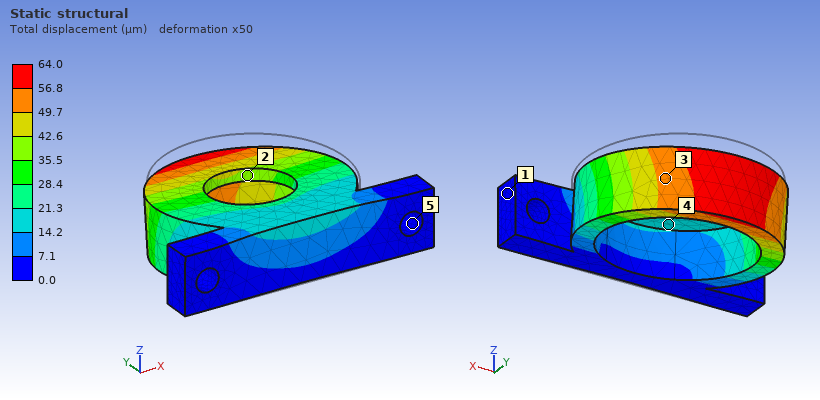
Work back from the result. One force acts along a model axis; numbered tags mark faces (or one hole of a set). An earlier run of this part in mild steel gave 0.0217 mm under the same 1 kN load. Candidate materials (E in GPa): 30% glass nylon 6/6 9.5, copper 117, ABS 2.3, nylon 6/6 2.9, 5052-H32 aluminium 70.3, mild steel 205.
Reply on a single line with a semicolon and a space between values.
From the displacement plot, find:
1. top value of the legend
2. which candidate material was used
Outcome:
64.0 µm; 5052-H32 aluminium
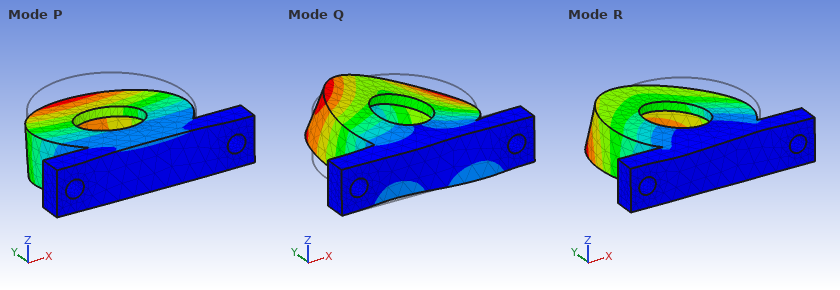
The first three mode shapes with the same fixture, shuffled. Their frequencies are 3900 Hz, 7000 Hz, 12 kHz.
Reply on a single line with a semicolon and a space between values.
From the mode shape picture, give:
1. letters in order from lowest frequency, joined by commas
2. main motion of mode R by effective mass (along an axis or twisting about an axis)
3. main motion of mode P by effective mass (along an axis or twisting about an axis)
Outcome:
P, R, Q; along X; along Z
